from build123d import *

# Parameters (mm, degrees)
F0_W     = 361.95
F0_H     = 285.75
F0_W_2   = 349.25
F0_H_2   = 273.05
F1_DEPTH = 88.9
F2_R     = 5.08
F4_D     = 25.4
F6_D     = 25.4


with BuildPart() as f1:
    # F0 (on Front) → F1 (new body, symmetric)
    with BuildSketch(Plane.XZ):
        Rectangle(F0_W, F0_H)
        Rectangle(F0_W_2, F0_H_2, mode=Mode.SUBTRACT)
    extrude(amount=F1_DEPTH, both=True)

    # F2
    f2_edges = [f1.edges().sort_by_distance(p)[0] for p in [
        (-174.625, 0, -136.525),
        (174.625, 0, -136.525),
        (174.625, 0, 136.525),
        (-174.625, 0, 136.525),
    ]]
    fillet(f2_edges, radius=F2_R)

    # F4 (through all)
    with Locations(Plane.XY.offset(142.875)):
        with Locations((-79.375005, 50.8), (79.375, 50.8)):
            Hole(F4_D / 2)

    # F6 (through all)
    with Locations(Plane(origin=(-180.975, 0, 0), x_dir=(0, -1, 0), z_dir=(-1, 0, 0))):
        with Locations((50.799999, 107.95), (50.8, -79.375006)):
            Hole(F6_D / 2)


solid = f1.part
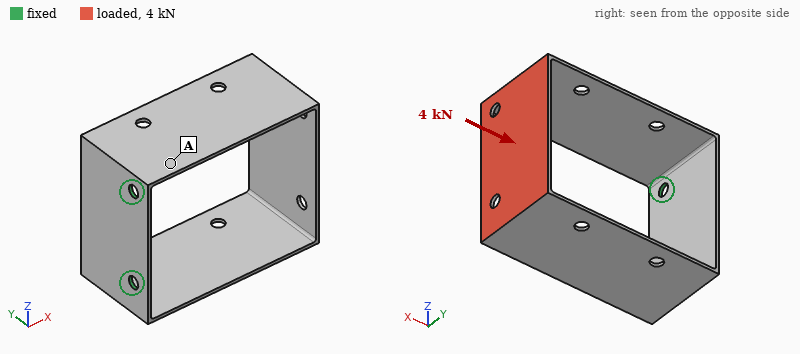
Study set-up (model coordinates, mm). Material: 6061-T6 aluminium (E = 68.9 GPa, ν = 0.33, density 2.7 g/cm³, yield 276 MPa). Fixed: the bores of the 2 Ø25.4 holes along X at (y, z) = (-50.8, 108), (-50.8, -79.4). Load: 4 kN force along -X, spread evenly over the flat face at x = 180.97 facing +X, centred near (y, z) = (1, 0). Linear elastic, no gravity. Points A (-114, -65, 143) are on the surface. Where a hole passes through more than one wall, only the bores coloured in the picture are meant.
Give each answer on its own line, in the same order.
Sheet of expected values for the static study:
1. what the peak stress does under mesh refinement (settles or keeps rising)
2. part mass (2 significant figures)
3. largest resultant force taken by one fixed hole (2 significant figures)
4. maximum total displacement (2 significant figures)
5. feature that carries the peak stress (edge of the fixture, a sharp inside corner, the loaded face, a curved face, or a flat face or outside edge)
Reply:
keeps rising
3.8 kg
2.1 kN
5.0 mm
edge of the fixture
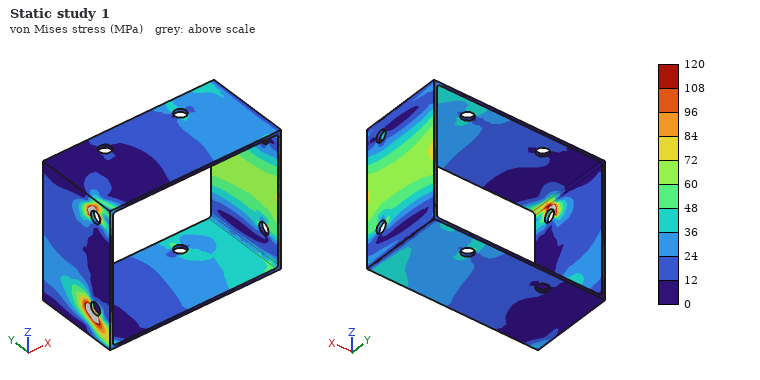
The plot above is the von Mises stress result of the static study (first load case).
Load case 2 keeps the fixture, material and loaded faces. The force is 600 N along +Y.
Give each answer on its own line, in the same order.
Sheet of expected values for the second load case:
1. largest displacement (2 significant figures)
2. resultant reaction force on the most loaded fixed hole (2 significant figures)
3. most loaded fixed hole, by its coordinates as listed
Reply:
4.0 mm
390 N
(-50.8, -79.4)
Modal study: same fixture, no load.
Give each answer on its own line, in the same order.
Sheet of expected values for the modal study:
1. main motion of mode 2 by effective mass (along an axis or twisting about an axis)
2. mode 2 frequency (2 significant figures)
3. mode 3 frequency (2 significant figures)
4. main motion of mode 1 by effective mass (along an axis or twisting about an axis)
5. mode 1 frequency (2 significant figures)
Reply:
along Y
53 Hz
97 Hz
along Z
35 Hz
